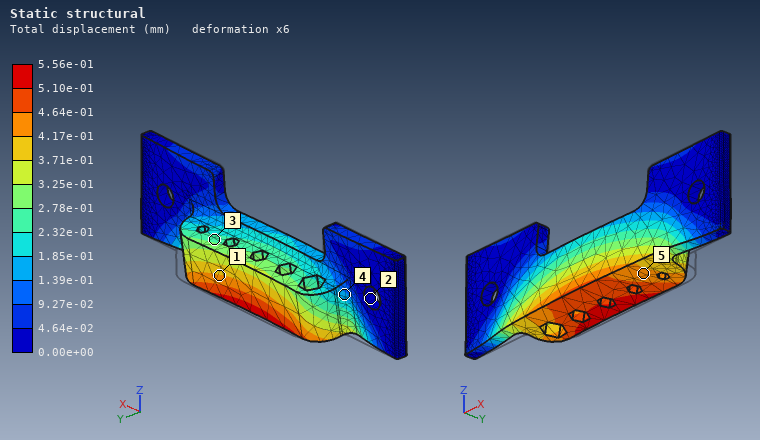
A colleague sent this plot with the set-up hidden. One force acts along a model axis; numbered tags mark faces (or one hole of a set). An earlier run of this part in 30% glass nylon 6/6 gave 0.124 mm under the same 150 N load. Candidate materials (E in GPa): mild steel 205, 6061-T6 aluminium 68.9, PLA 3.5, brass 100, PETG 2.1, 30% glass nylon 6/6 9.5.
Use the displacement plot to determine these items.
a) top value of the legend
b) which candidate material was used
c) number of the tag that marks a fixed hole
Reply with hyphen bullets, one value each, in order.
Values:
- 5.56e-01 mm
- PETG
- 2
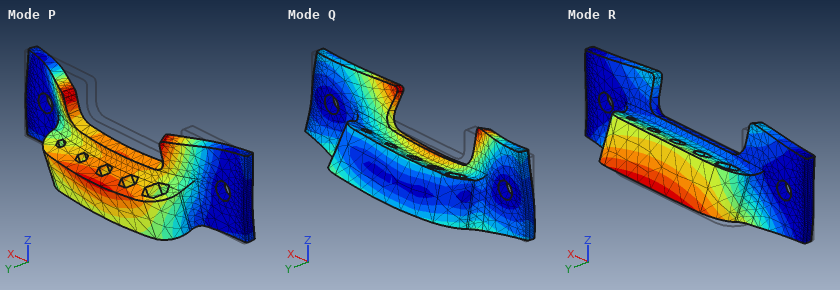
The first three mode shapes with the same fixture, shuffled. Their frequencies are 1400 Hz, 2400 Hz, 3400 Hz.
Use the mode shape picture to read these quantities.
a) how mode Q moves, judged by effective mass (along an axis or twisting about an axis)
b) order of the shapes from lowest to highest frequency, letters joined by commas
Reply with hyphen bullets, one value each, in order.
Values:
- along Z
- R, P, Q
